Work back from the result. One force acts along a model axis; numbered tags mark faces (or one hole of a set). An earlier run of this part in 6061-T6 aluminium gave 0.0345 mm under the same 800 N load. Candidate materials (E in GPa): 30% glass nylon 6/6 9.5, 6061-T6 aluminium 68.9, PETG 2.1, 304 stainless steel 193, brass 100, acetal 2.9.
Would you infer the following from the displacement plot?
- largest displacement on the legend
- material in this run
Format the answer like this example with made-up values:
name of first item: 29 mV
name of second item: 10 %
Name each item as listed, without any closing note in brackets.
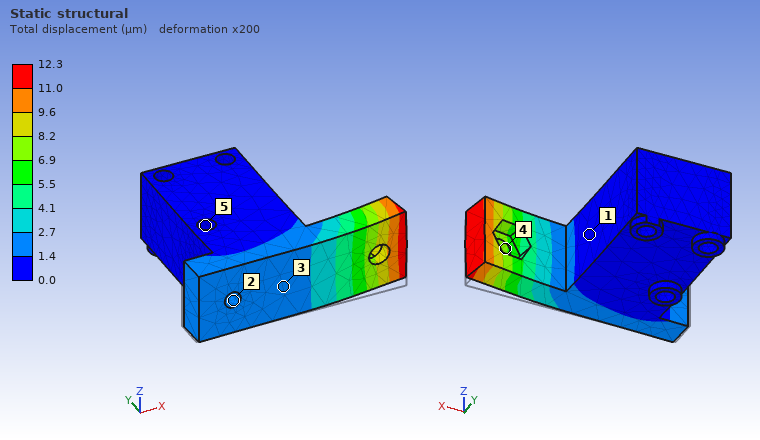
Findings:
largest displacement on the legend: 12.3 µm
material in this run: 304 stainless steel
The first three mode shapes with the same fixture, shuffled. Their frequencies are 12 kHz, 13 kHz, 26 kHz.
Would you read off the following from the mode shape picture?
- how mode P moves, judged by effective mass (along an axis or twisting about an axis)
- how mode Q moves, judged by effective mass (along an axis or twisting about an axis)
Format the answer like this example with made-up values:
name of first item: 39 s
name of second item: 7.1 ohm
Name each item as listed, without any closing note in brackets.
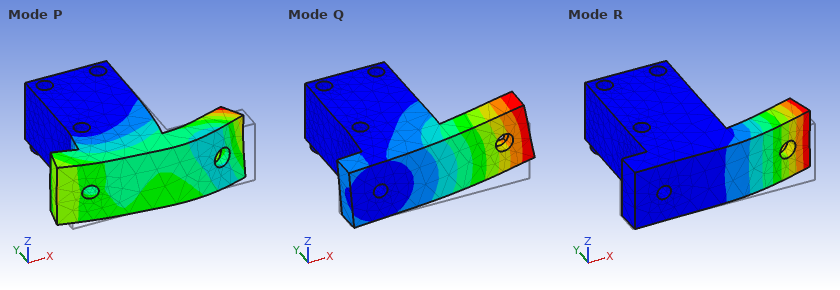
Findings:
how mode P moves, judged by effective mass: along X
how mode Q moves, judged by effective mass: along Z
